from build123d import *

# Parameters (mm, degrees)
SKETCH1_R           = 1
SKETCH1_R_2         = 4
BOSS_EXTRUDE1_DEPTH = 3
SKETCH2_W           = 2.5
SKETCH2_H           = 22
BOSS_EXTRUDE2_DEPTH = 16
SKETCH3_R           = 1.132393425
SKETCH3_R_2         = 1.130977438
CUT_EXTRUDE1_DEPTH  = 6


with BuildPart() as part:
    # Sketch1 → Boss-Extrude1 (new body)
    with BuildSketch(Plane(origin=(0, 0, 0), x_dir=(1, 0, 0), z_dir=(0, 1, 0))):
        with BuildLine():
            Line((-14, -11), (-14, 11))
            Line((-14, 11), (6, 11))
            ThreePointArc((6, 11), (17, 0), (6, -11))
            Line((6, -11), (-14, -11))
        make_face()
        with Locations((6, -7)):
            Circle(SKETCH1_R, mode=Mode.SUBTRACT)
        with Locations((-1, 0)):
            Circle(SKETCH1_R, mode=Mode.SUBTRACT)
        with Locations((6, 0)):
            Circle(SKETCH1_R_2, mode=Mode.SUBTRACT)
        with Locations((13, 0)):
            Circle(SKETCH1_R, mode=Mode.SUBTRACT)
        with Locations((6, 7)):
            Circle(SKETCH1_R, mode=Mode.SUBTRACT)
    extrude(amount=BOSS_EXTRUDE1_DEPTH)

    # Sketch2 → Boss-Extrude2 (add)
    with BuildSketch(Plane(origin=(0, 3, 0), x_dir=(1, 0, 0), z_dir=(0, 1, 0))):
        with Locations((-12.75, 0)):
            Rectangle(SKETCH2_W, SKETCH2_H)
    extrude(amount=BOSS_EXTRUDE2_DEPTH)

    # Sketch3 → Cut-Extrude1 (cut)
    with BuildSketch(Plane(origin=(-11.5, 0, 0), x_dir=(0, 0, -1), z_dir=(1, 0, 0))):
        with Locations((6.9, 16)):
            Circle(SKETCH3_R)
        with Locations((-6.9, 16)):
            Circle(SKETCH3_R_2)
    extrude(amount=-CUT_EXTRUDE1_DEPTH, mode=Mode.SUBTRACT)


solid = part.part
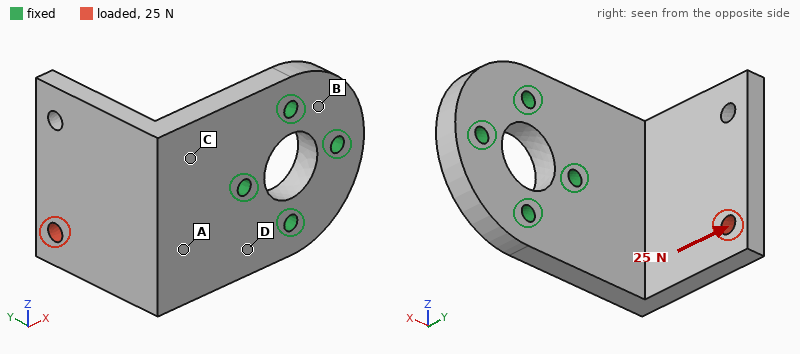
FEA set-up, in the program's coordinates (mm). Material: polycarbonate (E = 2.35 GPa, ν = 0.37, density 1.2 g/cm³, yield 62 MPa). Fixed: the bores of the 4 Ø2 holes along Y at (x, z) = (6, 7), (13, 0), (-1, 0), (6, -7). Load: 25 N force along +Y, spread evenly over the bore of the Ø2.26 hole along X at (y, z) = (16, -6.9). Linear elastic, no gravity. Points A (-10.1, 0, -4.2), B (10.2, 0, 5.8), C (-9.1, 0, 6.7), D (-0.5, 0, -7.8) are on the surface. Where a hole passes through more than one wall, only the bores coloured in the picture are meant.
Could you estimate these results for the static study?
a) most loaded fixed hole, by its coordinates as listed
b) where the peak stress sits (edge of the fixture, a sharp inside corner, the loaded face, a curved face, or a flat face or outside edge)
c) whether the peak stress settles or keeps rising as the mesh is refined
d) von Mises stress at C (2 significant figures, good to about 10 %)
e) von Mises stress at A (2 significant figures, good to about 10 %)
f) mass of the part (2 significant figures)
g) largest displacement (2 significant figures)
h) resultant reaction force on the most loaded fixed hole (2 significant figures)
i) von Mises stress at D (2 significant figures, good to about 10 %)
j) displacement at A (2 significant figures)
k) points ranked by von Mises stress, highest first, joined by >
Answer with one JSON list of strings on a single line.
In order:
["(-1, 0)", "edge of the fixture", "keeps rising", "4.7 MPa", "2.8 MPa", "3.1 g", "0.50 mm", "40 N", "6.3 MPa", "0.16 mm", "D > C > A > B"]
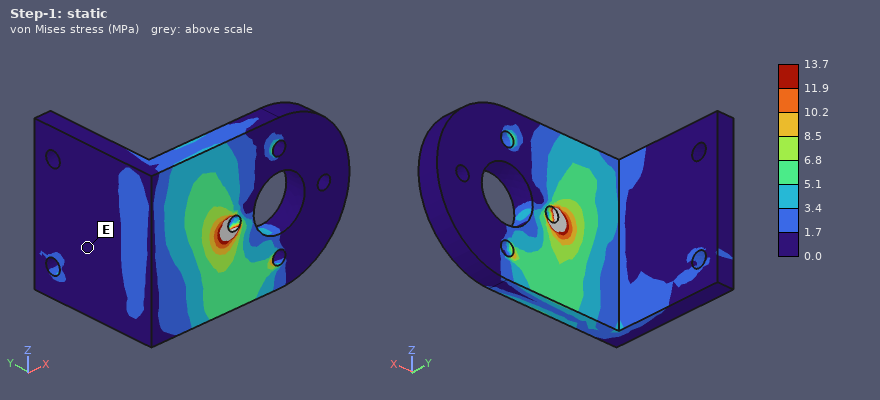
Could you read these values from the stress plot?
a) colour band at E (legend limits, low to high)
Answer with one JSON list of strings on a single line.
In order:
["0.0 to 1.7 MPa"]
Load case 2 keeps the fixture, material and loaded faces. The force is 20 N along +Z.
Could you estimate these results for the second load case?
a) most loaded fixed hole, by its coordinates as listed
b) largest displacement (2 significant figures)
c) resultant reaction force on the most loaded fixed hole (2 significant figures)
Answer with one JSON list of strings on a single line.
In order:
["(-1, 0)", "0.42 mm", "22 N"]
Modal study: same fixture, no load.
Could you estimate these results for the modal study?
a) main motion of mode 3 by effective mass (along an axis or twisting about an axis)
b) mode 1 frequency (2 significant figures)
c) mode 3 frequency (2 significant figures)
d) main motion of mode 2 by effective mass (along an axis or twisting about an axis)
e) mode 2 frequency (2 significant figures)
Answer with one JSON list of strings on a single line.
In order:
["along Y", "1100 Hz", "2600 Hz", "along Z", "1500 Hz"]
